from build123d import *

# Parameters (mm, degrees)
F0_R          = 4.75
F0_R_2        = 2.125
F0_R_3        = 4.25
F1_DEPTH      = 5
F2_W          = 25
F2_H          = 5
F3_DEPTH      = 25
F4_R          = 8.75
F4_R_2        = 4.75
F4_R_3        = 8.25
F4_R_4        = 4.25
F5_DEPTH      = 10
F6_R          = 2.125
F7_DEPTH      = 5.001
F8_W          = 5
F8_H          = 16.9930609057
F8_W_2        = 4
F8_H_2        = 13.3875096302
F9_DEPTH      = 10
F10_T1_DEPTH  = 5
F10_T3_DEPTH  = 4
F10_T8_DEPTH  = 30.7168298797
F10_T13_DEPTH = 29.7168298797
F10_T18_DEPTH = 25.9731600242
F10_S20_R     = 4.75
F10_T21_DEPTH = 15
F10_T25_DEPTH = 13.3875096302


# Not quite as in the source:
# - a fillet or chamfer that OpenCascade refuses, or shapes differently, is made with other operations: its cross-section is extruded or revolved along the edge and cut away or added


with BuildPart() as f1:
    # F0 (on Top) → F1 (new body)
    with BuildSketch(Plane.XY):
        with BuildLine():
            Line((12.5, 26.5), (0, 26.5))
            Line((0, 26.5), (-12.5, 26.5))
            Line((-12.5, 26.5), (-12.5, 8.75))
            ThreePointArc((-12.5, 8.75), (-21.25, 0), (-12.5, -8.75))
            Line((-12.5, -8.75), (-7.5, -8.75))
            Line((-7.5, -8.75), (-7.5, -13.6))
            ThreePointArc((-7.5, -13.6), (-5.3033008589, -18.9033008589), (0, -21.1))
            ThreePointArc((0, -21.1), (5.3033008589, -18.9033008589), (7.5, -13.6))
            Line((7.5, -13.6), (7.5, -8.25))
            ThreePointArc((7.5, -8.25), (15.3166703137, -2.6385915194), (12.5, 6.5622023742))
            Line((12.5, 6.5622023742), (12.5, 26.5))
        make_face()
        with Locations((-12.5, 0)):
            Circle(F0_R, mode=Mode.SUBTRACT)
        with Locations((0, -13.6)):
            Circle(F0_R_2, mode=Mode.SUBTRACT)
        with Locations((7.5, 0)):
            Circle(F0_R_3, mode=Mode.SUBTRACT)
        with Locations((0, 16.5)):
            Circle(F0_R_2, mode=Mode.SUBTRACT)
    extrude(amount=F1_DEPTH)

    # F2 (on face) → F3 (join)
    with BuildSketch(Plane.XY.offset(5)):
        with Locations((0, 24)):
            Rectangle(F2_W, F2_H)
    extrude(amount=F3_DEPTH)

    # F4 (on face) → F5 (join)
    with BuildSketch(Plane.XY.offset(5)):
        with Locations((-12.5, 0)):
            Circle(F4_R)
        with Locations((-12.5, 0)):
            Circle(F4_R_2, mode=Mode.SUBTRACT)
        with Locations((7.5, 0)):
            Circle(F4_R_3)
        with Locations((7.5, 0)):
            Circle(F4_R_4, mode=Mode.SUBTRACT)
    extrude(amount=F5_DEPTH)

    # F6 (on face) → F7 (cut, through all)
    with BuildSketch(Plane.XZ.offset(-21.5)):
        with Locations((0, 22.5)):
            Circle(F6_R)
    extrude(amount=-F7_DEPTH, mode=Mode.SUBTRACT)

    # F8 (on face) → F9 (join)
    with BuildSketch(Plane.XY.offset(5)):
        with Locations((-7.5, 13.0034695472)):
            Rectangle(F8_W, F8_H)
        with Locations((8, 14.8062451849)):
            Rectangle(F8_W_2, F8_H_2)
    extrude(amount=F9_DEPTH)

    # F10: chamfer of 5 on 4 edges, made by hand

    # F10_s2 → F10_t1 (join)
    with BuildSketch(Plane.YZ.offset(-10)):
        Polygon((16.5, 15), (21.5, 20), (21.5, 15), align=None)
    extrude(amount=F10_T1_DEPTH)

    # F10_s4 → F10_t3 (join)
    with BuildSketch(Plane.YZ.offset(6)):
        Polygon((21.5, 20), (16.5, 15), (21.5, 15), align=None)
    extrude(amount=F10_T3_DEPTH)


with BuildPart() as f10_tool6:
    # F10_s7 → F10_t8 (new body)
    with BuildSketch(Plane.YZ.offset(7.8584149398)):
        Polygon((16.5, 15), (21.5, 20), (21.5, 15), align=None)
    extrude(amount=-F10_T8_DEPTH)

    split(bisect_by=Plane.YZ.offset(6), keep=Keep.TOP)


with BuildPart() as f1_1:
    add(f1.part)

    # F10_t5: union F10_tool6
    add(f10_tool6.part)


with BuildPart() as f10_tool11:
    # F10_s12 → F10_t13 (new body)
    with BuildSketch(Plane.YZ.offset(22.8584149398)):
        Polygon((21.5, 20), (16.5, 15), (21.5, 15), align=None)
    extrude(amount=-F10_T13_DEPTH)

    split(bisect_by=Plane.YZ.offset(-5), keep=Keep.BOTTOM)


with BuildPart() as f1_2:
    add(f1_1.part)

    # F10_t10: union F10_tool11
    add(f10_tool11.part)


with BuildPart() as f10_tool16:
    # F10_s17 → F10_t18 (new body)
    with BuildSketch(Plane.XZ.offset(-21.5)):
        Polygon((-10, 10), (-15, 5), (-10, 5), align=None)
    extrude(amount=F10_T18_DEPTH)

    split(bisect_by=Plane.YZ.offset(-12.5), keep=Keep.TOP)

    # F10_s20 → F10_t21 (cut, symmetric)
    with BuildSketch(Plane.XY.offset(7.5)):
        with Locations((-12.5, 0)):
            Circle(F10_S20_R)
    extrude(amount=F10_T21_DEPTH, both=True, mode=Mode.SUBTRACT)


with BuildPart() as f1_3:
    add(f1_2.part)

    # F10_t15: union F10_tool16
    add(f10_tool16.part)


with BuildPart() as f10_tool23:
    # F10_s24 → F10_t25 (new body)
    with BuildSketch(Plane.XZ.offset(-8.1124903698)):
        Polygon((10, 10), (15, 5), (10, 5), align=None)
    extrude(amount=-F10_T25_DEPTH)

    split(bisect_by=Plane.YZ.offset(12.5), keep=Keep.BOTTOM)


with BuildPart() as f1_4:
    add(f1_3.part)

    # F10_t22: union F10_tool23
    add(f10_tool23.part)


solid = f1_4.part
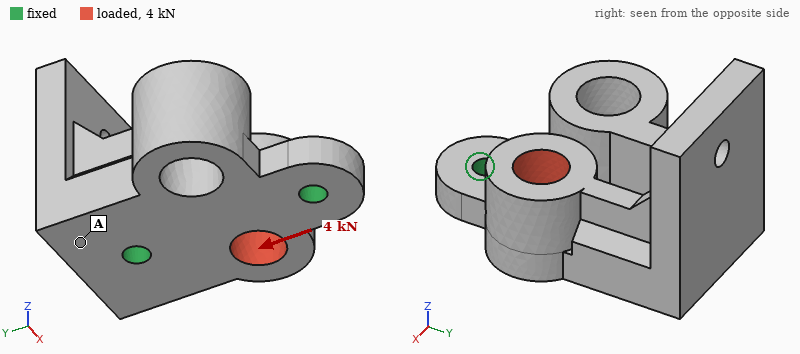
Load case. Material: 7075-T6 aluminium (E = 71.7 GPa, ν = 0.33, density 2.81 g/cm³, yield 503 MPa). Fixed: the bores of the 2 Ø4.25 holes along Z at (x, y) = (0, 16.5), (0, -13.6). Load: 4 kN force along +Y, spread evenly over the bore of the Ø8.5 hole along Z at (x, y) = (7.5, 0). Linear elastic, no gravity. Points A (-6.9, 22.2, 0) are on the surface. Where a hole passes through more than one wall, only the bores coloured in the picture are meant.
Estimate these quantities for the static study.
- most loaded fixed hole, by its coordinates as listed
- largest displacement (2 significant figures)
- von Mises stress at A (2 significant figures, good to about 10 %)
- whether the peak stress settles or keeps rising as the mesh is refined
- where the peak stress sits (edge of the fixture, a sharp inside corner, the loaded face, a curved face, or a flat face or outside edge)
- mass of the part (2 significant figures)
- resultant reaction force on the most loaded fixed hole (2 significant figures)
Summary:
(0, 16.5)
23 µm
15 MPa
keeps rising
edge of the fixture
37 g
2.5 kN
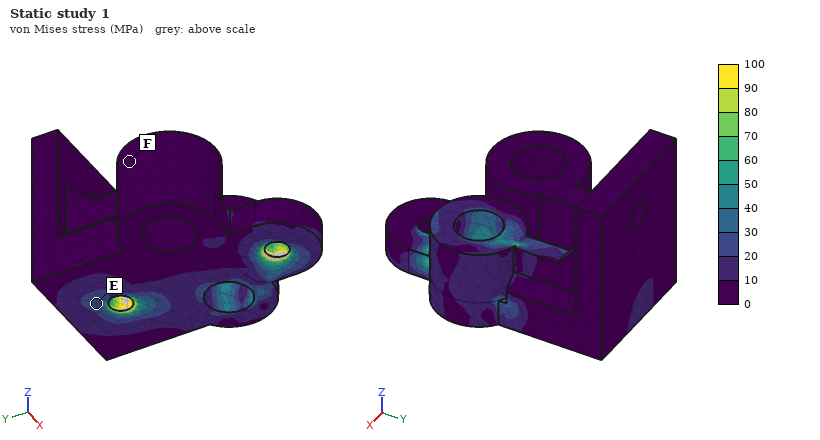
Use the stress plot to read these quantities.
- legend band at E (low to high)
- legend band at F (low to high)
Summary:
20 to 30 MPa
0 to 10 MPa
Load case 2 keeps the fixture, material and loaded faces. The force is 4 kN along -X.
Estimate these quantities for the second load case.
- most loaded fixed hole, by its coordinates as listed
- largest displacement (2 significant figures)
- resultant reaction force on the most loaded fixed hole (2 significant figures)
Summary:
(0, -13.6)
0.10 mm
2.2 kN
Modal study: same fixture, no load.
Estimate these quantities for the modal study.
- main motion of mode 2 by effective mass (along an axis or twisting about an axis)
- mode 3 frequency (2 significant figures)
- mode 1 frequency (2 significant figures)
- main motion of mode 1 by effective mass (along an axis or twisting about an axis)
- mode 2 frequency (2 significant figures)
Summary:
along Y
12 kHz
5600 Hz
along X
9200 Hz
